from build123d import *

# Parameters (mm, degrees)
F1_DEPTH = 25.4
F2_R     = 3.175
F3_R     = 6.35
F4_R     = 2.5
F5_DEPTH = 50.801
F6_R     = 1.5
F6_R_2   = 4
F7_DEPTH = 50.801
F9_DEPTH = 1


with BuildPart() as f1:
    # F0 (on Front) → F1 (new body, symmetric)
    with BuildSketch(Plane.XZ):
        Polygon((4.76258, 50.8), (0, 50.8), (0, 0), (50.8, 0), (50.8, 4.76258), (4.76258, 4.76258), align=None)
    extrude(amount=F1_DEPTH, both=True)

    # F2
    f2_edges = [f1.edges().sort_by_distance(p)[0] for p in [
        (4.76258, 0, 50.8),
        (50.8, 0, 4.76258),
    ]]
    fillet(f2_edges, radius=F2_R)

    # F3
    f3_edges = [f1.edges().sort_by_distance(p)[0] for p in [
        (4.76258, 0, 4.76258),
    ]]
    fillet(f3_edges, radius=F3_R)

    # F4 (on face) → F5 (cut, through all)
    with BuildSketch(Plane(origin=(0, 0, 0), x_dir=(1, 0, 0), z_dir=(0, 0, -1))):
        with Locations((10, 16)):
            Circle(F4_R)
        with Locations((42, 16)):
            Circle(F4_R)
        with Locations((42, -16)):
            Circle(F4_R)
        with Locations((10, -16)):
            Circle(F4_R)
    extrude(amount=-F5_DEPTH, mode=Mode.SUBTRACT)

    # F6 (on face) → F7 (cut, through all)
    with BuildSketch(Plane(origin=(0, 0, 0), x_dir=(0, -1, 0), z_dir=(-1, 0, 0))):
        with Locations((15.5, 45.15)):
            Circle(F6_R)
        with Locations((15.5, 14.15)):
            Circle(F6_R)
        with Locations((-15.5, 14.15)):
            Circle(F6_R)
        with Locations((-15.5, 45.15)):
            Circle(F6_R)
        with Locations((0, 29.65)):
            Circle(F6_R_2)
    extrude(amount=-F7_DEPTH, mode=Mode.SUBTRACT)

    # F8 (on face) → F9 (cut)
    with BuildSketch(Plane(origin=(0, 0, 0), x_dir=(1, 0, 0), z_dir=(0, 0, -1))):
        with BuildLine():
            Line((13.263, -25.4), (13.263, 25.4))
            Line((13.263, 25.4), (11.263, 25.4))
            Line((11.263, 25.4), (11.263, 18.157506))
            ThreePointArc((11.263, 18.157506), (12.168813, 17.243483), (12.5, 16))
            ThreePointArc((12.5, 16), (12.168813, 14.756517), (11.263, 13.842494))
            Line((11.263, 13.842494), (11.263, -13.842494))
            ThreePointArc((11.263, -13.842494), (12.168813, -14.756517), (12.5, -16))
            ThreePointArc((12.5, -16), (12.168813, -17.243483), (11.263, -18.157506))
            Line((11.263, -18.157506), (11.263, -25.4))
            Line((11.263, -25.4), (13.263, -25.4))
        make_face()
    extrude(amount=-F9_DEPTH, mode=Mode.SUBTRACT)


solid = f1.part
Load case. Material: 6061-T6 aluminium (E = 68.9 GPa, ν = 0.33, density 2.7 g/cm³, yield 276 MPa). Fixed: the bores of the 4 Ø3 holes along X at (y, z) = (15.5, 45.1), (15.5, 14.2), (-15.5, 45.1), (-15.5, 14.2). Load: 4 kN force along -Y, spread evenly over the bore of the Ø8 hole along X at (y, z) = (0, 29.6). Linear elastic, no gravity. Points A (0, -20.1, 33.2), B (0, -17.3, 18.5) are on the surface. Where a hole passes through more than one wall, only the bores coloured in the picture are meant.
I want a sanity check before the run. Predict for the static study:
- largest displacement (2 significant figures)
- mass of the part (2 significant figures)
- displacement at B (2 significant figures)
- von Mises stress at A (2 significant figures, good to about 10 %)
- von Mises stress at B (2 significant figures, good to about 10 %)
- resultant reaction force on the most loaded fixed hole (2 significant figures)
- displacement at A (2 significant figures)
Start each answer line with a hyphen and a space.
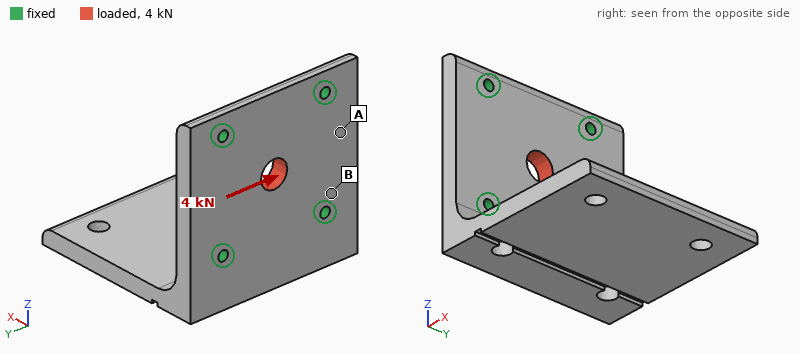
- 7.9 µm
- 62 g
- 2.0 µm
- 7.6 MPa
- 15 MPa
- 1.1 kN
- 4.1 µm
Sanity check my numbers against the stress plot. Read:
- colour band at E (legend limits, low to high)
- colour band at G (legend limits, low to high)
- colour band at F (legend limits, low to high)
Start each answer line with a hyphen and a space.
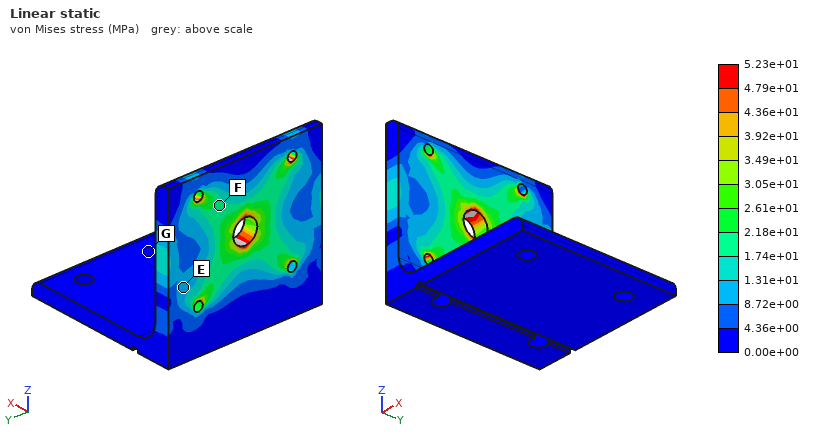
- 8.72e+00 to 1.31e+01 MPa
- 0.00e+00 to 4.36e+00 MPa
- 1.74e+01 to 2.18e+01 MPa
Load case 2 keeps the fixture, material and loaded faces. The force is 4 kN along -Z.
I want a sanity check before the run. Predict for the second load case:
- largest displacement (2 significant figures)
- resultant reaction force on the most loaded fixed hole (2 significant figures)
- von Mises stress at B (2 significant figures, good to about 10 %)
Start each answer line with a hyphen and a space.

- 8.4 µm
- 1.1 kN
- 8.8 MPa
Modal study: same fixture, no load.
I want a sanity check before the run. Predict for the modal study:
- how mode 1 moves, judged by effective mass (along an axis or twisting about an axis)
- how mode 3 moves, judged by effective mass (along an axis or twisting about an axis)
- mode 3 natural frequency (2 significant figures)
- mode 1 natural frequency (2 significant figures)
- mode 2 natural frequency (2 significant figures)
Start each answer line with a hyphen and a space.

- along Z
- along Y
- 4700 Hz
- 1300 Hz
- 3300 Hz
